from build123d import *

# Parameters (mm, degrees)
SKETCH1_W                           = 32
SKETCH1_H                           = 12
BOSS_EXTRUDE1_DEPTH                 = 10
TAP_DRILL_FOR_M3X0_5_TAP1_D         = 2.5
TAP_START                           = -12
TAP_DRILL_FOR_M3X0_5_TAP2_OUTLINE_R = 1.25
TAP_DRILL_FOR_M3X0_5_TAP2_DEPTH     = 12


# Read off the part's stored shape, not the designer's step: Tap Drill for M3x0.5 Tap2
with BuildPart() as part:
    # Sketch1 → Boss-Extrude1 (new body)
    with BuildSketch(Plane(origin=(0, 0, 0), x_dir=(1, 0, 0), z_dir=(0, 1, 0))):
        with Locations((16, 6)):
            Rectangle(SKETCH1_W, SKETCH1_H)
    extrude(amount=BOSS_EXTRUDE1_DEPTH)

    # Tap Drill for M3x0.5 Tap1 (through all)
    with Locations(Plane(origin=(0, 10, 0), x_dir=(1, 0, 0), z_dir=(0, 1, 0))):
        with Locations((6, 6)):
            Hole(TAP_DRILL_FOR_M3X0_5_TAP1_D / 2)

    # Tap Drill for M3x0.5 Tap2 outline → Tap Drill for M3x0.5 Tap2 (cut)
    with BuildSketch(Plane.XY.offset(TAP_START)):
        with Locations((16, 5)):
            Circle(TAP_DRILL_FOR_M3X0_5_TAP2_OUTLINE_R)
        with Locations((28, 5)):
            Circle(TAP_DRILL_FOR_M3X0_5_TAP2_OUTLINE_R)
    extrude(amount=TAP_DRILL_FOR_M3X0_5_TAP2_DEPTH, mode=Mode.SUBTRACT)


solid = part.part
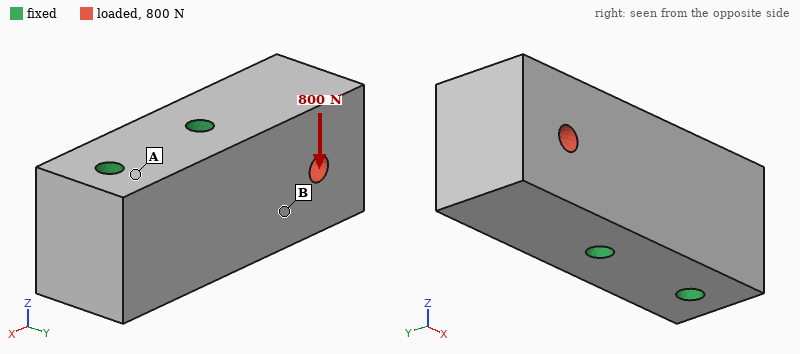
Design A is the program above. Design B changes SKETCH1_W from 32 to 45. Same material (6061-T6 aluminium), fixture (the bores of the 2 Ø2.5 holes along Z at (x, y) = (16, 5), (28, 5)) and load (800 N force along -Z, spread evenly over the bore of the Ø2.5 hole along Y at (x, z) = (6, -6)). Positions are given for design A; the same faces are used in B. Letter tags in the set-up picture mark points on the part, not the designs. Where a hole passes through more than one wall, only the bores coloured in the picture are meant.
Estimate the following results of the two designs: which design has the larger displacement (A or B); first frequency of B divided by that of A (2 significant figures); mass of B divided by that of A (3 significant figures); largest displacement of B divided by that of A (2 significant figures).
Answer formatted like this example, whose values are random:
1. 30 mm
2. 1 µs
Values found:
1. B
2. 0.57
3. 1.42
4. 1.3
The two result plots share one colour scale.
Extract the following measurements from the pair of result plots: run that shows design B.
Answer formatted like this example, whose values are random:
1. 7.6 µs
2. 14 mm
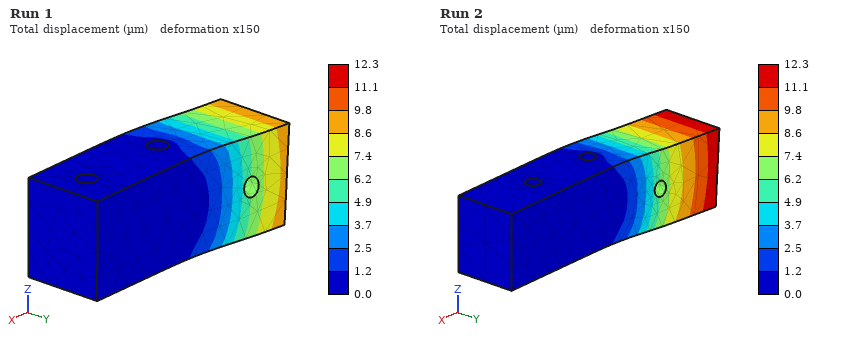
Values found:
1. Run 2
